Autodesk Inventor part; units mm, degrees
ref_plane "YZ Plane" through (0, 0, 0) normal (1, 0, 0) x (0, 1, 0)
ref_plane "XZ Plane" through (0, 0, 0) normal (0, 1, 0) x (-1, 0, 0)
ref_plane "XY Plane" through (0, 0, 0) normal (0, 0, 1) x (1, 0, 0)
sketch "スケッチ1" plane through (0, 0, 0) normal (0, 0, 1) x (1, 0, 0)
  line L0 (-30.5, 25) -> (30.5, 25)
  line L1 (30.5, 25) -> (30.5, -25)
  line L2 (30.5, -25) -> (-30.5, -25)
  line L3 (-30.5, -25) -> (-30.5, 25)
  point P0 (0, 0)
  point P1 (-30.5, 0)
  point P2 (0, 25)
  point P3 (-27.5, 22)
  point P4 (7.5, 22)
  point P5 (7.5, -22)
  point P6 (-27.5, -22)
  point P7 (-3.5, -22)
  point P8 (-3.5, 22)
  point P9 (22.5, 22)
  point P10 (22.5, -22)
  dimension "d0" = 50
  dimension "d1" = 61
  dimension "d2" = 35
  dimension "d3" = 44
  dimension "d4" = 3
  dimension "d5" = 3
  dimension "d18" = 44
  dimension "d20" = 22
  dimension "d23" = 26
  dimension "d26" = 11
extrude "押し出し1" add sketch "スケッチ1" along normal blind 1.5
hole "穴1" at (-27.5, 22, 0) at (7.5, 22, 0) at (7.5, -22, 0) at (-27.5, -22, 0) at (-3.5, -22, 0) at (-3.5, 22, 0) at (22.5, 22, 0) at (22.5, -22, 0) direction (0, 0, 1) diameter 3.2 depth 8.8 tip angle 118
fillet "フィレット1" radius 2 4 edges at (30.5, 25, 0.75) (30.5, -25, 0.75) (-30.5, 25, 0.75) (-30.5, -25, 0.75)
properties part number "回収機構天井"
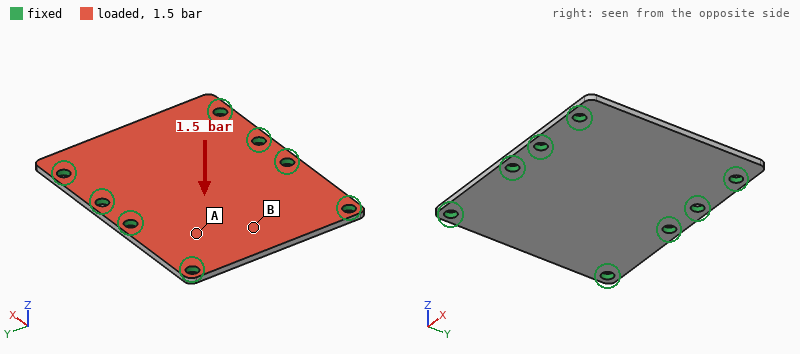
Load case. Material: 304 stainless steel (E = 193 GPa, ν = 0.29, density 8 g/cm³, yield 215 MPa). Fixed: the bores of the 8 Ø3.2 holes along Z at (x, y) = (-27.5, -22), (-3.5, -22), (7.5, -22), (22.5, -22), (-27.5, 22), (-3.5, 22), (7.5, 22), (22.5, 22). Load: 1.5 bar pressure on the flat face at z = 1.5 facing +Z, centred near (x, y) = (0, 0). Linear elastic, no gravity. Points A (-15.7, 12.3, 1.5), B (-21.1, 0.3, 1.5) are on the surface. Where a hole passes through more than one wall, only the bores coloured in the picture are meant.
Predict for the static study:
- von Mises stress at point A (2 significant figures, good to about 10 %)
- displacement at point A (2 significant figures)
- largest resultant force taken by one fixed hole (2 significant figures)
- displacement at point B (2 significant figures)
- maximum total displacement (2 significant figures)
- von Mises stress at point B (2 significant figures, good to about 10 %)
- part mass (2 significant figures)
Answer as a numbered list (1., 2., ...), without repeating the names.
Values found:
1. 12 MPa
2. 16 µm
3. 66 N
4. 29 µm
5. 29 µm
6. 29 MPa
7. 36 g
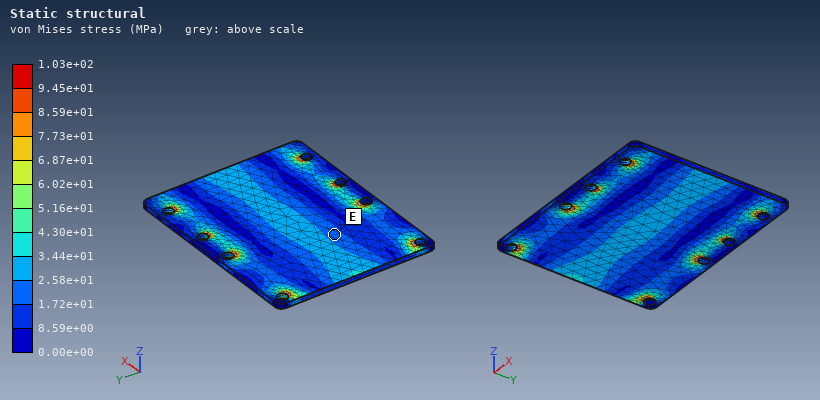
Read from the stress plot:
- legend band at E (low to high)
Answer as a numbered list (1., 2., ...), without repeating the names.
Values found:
1. 1.72e+01 to 2.58e+01 MPa
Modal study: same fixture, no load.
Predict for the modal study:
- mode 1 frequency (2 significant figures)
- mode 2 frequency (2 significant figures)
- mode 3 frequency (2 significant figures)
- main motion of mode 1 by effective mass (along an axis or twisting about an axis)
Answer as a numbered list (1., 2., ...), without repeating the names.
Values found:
1. 3900 Hz
2. 4400 Hz
3. 6100 Hz
4. along Z
